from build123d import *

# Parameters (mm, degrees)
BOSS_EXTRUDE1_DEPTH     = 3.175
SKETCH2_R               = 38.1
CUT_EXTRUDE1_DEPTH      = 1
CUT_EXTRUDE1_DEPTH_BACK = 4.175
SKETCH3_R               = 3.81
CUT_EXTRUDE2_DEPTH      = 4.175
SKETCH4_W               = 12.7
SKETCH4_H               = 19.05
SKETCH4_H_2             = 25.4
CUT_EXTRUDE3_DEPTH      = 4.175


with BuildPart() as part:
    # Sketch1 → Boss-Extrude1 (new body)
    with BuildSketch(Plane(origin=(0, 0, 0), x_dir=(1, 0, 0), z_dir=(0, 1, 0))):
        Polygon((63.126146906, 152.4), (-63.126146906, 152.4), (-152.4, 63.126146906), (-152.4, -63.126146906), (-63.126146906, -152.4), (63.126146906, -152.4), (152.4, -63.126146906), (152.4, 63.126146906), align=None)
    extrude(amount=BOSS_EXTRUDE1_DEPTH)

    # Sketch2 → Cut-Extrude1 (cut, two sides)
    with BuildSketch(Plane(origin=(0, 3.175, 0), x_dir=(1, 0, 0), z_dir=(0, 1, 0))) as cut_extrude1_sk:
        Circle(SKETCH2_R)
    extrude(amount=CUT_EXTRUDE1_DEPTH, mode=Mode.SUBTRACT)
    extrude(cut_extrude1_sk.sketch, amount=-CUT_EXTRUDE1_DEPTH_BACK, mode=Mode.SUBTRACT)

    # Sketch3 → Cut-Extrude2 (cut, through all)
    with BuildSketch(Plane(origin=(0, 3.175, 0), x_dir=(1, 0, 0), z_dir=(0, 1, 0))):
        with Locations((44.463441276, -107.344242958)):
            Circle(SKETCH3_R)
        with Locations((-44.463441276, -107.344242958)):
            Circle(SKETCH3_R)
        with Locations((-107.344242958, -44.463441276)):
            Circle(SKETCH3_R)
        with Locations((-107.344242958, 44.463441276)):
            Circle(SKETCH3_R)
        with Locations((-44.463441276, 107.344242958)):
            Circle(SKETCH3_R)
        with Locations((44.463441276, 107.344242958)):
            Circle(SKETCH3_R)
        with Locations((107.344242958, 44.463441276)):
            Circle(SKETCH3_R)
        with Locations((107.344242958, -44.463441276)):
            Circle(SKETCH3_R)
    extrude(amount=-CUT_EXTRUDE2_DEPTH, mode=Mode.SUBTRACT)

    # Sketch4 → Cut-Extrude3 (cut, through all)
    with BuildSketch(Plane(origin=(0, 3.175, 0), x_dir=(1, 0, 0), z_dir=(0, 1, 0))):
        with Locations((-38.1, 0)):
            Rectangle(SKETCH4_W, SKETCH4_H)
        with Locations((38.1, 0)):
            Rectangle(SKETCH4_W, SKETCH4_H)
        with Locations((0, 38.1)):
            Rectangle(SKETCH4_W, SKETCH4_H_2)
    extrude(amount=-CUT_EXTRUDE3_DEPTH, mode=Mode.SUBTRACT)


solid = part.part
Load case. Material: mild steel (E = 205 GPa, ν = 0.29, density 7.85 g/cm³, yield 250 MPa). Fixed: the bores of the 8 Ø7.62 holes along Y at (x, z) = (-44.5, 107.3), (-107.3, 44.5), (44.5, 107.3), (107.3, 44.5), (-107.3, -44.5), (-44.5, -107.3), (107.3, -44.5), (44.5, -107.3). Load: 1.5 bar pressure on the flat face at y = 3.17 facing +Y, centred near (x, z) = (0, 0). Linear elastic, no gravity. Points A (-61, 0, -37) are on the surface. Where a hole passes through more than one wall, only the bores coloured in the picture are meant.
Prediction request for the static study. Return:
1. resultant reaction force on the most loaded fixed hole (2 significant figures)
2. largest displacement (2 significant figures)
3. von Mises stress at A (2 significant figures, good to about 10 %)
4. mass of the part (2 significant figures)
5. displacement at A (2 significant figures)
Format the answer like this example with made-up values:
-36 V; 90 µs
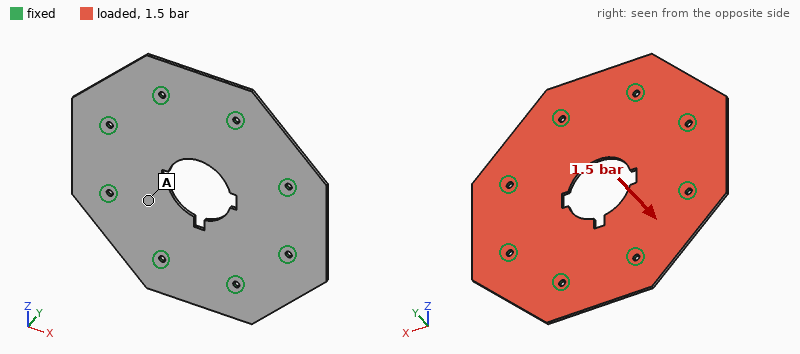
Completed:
1.3 kN; 0.61 mm; 39 MPa; 1.8 kg; 0.28 mm
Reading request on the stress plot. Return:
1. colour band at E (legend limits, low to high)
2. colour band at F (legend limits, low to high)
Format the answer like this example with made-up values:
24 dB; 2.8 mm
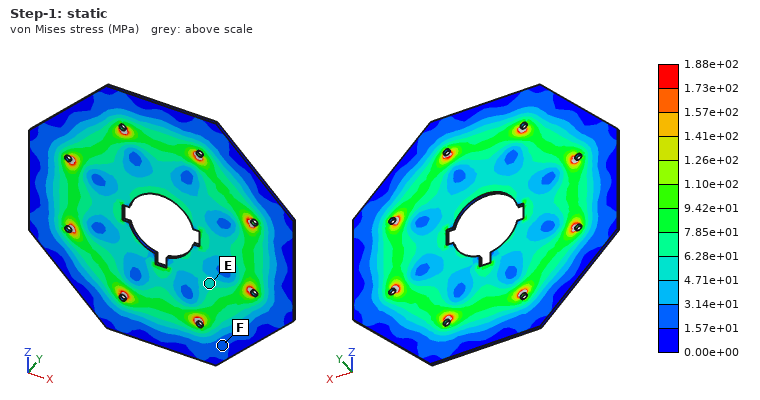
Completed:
4.71e+01 to 6.28e+01 MPa; 1.57e+01 to 3.14e+01 MPa
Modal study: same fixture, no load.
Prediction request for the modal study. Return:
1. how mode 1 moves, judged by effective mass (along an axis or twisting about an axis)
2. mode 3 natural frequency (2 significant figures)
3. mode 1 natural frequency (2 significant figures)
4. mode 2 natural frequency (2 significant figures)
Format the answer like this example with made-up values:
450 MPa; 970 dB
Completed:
along Y; 950 Hz; 610 Hz; 940 Hz
